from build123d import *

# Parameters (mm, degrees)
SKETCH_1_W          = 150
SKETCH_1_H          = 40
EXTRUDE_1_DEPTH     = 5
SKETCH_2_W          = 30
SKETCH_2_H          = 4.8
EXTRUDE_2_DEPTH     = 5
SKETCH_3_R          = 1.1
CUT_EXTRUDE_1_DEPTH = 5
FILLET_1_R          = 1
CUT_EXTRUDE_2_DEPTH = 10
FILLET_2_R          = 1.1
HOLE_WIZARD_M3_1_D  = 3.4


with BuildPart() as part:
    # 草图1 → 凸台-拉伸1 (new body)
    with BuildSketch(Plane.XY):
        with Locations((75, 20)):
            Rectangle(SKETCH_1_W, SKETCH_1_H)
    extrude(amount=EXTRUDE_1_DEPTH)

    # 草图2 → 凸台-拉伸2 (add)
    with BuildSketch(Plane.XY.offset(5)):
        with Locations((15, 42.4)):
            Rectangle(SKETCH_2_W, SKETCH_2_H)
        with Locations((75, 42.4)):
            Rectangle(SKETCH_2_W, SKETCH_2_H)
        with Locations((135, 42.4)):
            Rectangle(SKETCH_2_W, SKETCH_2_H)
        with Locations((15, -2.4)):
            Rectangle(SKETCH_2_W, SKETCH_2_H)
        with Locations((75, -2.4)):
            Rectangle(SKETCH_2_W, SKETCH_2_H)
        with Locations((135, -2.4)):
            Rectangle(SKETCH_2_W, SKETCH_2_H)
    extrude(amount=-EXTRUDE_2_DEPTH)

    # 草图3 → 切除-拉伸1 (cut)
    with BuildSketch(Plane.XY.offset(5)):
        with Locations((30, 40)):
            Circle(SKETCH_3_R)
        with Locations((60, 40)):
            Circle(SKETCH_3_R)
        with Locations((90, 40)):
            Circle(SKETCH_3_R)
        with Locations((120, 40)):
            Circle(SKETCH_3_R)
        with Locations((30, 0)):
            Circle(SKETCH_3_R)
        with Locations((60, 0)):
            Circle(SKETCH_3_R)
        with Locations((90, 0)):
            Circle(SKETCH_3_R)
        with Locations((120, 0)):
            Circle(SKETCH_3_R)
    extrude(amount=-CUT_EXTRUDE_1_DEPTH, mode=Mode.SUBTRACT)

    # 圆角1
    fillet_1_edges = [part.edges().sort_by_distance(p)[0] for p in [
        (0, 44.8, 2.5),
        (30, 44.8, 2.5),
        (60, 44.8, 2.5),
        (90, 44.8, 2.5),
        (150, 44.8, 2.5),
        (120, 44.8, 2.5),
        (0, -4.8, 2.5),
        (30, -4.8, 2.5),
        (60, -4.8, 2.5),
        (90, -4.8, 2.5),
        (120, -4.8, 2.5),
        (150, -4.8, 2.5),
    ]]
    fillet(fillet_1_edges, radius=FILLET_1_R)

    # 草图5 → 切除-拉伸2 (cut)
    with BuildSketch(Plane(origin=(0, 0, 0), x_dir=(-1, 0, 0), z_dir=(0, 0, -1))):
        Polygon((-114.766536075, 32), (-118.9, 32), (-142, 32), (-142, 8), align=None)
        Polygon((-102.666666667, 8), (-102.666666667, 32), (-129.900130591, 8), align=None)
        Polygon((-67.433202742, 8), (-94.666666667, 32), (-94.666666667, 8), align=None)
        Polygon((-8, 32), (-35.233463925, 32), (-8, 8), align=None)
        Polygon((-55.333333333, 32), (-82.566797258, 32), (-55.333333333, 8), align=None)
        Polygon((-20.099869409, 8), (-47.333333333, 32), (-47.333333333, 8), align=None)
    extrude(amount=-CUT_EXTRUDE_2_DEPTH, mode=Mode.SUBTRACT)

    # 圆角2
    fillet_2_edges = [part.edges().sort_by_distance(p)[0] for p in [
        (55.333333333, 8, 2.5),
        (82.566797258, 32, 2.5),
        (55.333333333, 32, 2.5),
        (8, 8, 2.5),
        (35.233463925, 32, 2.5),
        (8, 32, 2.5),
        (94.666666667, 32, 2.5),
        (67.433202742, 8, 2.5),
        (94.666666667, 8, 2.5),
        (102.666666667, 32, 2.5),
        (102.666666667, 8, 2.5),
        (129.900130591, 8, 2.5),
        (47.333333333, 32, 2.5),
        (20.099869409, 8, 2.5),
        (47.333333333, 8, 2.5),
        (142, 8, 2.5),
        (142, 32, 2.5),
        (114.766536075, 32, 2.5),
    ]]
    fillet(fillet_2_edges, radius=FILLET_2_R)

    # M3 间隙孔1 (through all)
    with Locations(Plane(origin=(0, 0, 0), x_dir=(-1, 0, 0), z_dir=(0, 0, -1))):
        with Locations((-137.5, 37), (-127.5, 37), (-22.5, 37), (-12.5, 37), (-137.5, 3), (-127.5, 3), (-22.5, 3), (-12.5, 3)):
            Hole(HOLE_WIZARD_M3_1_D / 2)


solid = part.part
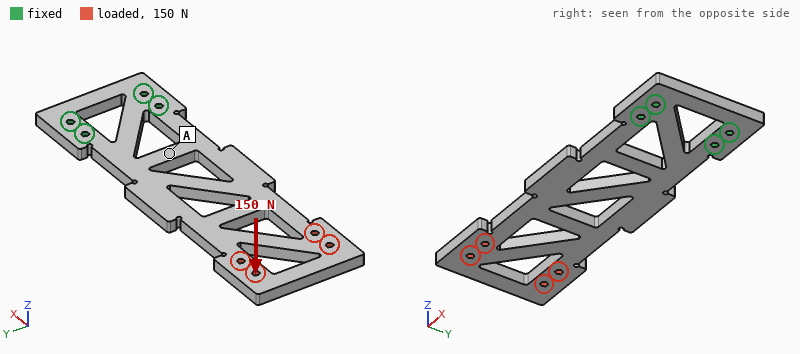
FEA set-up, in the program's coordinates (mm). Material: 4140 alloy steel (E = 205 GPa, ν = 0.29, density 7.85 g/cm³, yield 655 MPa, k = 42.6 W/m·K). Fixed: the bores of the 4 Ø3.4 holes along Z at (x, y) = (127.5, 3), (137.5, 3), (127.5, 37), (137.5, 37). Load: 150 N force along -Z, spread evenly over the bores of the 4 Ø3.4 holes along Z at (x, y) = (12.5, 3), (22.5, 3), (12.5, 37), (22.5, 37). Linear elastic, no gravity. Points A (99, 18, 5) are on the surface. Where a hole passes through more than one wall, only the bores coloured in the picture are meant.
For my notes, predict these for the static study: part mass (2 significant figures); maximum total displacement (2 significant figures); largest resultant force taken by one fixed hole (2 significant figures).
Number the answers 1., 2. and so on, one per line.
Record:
1. 190 g
2. 1.8 mm
3. 390 N
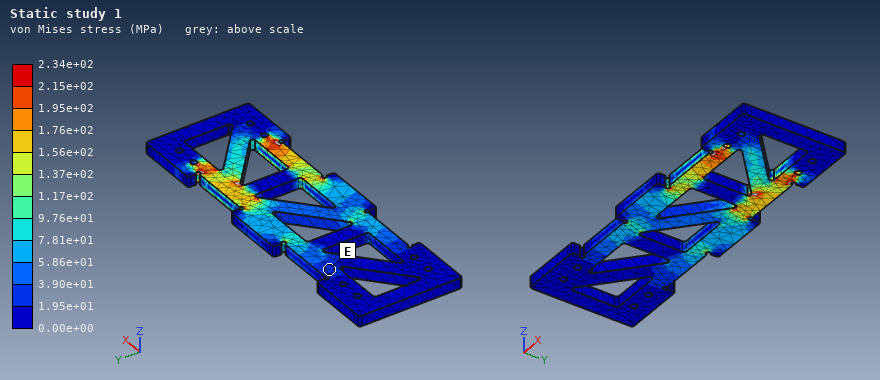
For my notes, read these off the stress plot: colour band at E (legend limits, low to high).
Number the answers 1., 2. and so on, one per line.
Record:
1. 1.95e+01 to 3.90e+01 MPa
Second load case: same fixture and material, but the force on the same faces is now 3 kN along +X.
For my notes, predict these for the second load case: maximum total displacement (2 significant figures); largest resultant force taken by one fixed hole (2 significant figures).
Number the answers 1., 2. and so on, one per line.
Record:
1. 21 µm
2. 1.3 kN
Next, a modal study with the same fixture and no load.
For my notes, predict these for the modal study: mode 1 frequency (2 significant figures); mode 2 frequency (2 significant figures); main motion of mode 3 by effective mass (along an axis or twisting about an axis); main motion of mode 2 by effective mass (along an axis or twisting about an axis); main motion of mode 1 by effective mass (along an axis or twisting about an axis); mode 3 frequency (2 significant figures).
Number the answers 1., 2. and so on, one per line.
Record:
1. 200 Hz
2. 1000 Hz
3. along Z
4. twisting about X
5. along Z
6. 1300 Hz
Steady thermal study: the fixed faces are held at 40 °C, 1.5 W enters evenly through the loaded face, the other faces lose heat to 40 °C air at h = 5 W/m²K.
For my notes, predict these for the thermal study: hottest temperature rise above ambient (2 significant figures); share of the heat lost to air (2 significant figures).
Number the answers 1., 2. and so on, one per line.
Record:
1. 23 K
2. 49 %
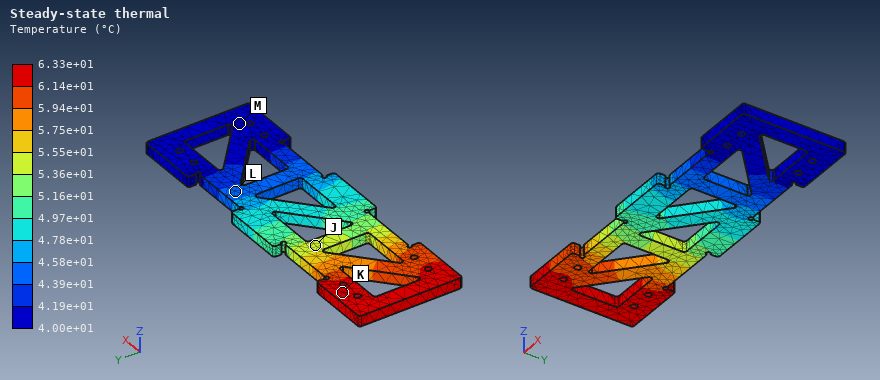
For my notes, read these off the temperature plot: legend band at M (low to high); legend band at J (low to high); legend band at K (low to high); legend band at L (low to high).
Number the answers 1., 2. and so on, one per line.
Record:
1. 4.00e+01 to 4.19e+01 °C
2. 5.36e+01 to 5.55e+01 °C
3. 6.14e+01 to 6.33e+01 °C
4. 4.39e+01 to 4.58e+01 °C
